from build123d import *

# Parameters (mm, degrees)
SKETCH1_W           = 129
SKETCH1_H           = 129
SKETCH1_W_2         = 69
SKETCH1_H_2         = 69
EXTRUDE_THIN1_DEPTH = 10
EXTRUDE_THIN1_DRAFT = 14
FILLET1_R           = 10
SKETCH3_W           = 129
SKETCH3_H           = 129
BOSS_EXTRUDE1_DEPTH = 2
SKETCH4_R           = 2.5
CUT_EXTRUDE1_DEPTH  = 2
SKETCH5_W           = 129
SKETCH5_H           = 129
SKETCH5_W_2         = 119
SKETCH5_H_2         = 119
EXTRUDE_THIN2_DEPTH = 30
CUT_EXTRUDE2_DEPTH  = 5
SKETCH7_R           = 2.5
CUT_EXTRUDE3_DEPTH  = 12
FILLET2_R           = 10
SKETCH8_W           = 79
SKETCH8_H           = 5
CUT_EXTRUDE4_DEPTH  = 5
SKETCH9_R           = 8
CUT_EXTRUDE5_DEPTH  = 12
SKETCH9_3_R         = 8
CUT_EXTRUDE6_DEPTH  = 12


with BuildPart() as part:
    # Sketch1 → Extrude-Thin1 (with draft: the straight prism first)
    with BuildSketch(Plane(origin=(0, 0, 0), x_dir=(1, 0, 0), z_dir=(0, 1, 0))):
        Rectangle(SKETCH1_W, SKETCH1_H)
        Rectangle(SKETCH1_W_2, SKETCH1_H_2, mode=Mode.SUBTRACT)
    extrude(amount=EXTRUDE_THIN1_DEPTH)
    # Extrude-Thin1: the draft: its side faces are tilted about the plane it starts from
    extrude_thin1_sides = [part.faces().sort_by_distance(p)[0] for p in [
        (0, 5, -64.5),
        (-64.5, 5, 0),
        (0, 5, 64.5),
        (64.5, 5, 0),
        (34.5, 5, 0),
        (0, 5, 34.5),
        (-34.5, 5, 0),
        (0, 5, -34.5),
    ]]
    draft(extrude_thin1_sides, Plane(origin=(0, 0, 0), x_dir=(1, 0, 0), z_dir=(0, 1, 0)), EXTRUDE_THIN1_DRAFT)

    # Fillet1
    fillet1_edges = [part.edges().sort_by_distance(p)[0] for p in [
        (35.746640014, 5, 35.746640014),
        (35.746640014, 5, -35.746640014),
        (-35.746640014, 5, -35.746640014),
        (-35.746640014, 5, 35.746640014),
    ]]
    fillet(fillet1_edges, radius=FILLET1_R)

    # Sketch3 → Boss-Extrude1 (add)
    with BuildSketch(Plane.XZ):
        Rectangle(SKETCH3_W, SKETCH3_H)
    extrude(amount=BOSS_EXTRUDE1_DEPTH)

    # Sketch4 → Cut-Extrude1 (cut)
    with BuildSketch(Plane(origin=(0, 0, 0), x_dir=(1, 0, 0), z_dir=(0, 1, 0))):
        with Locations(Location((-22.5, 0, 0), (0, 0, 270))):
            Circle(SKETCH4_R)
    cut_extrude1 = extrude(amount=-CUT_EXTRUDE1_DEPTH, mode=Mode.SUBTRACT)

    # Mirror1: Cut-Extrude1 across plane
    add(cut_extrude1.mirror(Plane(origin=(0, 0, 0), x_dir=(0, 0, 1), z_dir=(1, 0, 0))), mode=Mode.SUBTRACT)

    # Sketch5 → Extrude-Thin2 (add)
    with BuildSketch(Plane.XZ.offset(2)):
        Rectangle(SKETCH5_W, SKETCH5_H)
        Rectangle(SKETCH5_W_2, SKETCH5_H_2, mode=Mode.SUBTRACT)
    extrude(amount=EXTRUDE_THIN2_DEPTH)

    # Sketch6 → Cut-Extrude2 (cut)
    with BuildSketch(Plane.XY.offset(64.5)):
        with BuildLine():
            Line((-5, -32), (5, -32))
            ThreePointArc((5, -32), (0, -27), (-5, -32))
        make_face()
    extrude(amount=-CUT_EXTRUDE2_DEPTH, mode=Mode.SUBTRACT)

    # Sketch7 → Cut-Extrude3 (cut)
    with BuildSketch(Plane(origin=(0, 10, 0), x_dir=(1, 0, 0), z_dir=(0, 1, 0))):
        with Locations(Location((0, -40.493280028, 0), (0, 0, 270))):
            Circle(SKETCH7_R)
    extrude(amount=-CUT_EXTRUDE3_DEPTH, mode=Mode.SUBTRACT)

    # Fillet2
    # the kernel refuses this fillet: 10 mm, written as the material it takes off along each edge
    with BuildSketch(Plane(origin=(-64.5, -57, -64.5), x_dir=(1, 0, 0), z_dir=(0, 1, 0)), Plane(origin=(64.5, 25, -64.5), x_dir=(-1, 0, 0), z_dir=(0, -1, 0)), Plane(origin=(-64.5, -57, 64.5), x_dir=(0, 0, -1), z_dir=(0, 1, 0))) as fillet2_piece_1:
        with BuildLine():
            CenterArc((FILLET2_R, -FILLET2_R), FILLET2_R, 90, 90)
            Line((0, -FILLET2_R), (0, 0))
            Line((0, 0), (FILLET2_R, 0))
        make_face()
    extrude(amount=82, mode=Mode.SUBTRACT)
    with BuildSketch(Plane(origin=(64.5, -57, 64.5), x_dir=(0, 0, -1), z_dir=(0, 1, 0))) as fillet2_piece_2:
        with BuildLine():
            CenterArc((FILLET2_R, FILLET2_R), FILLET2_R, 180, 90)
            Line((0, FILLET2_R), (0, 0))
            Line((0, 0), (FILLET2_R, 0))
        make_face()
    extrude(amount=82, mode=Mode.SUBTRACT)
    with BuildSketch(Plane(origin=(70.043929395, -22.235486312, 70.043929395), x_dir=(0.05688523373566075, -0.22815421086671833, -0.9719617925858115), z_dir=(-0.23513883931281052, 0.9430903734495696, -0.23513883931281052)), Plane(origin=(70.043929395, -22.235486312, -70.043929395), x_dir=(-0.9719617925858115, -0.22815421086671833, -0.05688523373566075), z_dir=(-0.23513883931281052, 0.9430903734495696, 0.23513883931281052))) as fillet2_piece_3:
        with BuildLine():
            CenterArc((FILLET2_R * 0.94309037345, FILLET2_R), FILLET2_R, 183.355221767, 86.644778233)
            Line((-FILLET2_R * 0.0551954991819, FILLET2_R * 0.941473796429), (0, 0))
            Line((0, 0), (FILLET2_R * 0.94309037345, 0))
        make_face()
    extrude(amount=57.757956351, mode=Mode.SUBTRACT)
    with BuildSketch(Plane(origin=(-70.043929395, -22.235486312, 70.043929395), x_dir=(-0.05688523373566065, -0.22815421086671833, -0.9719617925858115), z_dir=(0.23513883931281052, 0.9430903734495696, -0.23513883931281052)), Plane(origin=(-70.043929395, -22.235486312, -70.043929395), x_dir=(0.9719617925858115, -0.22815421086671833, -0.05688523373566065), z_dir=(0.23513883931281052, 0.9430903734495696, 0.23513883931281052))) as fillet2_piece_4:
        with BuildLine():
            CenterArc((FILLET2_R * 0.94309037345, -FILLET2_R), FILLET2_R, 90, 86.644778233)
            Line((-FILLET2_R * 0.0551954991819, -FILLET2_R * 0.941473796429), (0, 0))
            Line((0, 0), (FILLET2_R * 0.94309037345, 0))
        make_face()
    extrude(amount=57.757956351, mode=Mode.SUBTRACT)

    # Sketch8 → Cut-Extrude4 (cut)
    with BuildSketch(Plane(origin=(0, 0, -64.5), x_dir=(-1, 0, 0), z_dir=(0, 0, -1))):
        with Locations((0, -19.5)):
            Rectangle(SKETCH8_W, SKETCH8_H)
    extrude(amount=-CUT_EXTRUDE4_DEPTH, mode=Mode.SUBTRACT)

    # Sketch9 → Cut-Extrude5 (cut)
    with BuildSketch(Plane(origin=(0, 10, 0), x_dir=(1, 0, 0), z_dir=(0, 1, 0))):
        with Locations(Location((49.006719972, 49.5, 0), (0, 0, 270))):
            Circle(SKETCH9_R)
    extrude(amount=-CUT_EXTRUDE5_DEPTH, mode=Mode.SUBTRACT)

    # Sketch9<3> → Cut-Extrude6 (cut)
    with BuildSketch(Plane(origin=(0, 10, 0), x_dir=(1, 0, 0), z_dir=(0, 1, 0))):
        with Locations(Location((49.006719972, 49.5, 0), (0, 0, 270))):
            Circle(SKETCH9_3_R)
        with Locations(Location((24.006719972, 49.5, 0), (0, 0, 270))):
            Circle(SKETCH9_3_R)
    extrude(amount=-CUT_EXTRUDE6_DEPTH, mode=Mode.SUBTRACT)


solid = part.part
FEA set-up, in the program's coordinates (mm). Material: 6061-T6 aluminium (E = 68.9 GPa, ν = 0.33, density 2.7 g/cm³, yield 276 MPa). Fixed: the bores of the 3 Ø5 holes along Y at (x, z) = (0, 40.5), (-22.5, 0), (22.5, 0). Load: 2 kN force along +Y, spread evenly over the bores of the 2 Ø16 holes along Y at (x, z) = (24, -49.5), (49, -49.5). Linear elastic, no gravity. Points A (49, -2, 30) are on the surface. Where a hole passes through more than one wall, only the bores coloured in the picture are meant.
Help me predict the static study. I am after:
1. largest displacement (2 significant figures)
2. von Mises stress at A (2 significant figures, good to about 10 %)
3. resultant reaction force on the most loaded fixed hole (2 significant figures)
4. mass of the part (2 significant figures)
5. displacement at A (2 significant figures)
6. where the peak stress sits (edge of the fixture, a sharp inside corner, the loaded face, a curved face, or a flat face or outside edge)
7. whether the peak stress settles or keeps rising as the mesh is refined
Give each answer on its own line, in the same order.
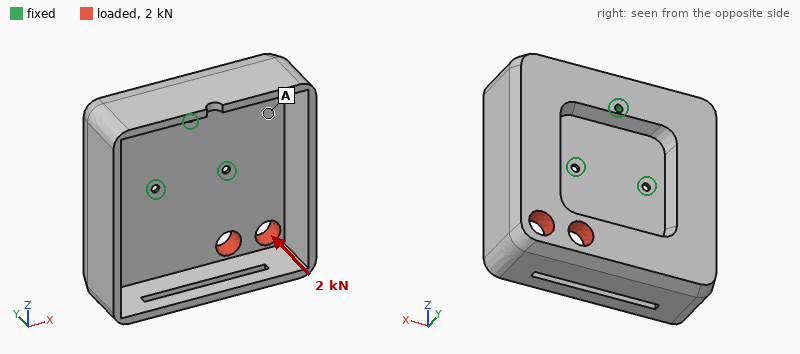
0.94 mm
37 MPa
3.3 kN
560 g
0.18 mm
edge of the fixture
keeps rising
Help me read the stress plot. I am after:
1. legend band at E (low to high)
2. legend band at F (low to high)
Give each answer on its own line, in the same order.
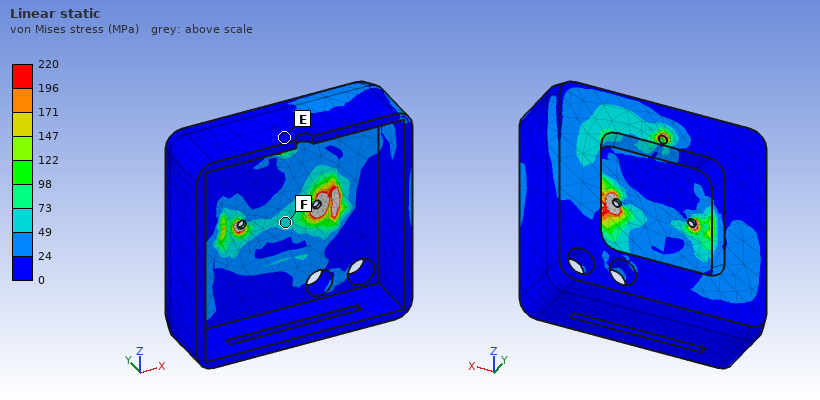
0 to 24 MPa
49 to 73 MPa
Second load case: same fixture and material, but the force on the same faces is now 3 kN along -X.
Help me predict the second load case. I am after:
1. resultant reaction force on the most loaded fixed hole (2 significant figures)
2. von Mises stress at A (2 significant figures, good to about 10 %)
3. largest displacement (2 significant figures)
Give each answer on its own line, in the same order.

2.9 kN
12 MPa
0.11 mm
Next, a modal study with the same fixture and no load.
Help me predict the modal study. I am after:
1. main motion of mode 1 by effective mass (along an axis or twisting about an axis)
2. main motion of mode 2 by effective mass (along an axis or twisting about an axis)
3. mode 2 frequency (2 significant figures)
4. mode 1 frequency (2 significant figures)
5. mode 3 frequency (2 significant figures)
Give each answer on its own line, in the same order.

along Y
twisting about Z
770 Hz
660 Hz
1500 Hz
